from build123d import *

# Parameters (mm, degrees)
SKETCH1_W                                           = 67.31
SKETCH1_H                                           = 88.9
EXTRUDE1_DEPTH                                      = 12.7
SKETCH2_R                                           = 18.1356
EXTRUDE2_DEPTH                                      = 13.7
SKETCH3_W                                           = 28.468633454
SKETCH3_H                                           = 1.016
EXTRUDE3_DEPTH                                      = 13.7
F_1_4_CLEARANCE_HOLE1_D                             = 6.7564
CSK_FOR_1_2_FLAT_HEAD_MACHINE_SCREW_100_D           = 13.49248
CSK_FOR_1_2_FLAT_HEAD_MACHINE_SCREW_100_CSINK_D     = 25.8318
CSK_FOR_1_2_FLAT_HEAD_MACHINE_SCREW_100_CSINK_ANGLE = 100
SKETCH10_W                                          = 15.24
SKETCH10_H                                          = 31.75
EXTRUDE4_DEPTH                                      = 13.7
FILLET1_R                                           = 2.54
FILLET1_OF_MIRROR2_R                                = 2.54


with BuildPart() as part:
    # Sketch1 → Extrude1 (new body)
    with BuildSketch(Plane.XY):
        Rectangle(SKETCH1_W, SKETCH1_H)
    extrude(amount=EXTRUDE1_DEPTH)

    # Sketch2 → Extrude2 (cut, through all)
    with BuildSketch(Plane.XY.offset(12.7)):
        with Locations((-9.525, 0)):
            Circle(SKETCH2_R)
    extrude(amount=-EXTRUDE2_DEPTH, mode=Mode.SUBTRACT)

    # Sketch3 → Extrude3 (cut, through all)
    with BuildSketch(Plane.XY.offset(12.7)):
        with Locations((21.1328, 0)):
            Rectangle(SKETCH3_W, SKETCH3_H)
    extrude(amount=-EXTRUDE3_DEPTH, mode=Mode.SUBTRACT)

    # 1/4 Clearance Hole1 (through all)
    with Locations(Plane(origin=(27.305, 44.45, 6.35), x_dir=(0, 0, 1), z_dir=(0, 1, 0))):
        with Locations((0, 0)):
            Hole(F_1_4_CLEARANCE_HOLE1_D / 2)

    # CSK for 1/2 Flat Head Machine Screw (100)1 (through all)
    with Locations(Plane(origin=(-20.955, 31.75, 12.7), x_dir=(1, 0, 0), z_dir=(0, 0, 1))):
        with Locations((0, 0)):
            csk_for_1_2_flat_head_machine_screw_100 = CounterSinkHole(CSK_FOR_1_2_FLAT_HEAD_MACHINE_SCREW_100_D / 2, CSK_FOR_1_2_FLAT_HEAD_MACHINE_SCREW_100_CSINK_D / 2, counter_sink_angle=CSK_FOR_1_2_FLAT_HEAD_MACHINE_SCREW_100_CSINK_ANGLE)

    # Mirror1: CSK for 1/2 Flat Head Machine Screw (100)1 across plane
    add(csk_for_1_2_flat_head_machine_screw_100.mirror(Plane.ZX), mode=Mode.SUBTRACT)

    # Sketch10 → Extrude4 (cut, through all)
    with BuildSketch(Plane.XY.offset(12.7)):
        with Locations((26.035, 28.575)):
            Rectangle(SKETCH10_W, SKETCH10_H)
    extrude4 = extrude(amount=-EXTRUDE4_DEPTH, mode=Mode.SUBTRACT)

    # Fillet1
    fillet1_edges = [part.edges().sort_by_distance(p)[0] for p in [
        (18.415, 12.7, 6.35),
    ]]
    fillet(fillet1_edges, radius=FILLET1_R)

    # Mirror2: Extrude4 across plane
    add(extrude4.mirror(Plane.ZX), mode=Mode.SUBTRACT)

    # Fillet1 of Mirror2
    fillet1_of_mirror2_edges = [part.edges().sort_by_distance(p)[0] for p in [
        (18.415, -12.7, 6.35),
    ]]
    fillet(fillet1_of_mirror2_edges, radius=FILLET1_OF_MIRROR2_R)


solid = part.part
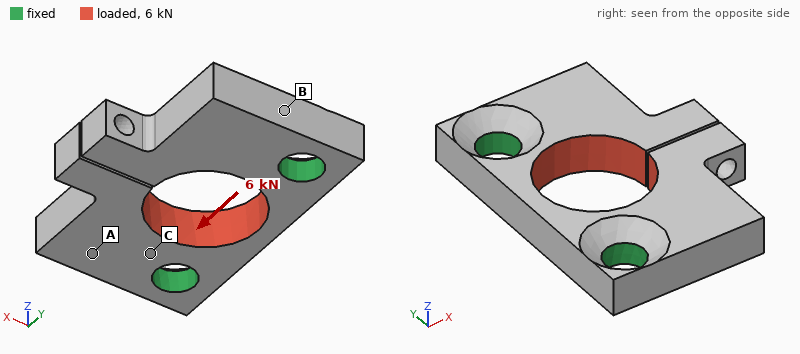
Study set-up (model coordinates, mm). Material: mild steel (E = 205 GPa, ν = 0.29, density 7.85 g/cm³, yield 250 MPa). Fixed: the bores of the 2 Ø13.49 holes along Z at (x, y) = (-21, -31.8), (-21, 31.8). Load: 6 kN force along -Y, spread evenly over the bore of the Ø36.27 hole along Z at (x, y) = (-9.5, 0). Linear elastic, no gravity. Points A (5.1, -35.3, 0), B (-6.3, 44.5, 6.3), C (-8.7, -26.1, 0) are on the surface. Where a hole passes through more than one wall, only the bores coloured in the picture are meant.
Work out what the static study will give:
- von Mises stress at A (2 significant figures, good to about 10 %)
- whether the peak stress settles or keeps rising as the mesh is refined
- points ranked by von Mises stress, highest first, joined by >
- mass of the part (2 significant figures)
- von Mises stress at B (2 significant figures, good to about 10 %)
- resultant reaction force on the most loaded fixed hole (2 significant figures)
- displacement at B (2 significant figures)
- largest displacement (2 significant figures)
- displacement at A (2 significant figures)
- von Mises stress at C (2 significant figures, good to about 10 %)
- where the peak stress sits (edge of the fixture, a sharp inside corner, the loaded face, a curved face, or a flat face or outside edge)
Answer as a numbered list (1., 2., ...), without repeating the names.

1. 3.5 MPa
2. keeps rising
3. C > B > A
4. 350 g
5. 8.1 MPa
6. 3.0 kN
7. 2.4 µm
8. 8.0 µm
9. 3.5 µm
10. 13 MPa
11. edge of the fixture
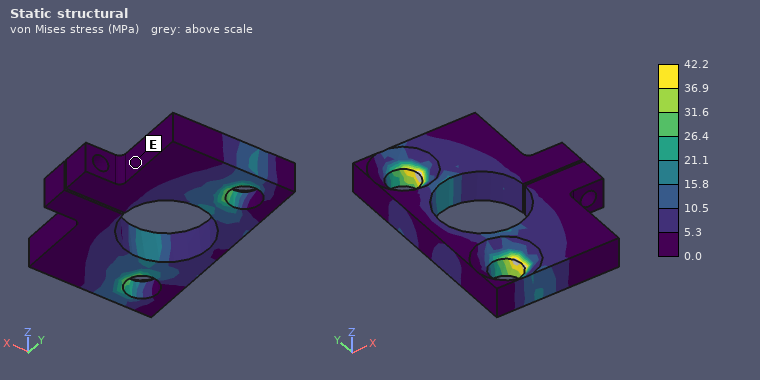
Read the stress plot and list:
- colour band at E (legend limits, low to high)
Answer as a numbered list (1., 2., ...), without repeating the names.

1. 0.0 to 5.3 MPa
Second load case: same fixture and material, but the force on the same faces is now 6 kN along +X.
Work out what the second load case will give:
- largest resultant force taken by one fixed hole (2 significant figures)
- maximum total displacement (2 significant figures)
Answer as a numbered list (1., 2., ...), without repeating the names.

1. 3.1 kN
2. 19 µm
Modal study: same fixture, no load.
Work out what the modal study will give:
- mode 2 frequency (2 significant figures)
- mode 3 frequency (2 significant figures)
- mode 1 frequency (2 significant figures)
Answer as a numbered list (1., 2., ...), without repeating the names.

1. 3400 Hz
2. 5800 Hz
3. 3400 Hz
